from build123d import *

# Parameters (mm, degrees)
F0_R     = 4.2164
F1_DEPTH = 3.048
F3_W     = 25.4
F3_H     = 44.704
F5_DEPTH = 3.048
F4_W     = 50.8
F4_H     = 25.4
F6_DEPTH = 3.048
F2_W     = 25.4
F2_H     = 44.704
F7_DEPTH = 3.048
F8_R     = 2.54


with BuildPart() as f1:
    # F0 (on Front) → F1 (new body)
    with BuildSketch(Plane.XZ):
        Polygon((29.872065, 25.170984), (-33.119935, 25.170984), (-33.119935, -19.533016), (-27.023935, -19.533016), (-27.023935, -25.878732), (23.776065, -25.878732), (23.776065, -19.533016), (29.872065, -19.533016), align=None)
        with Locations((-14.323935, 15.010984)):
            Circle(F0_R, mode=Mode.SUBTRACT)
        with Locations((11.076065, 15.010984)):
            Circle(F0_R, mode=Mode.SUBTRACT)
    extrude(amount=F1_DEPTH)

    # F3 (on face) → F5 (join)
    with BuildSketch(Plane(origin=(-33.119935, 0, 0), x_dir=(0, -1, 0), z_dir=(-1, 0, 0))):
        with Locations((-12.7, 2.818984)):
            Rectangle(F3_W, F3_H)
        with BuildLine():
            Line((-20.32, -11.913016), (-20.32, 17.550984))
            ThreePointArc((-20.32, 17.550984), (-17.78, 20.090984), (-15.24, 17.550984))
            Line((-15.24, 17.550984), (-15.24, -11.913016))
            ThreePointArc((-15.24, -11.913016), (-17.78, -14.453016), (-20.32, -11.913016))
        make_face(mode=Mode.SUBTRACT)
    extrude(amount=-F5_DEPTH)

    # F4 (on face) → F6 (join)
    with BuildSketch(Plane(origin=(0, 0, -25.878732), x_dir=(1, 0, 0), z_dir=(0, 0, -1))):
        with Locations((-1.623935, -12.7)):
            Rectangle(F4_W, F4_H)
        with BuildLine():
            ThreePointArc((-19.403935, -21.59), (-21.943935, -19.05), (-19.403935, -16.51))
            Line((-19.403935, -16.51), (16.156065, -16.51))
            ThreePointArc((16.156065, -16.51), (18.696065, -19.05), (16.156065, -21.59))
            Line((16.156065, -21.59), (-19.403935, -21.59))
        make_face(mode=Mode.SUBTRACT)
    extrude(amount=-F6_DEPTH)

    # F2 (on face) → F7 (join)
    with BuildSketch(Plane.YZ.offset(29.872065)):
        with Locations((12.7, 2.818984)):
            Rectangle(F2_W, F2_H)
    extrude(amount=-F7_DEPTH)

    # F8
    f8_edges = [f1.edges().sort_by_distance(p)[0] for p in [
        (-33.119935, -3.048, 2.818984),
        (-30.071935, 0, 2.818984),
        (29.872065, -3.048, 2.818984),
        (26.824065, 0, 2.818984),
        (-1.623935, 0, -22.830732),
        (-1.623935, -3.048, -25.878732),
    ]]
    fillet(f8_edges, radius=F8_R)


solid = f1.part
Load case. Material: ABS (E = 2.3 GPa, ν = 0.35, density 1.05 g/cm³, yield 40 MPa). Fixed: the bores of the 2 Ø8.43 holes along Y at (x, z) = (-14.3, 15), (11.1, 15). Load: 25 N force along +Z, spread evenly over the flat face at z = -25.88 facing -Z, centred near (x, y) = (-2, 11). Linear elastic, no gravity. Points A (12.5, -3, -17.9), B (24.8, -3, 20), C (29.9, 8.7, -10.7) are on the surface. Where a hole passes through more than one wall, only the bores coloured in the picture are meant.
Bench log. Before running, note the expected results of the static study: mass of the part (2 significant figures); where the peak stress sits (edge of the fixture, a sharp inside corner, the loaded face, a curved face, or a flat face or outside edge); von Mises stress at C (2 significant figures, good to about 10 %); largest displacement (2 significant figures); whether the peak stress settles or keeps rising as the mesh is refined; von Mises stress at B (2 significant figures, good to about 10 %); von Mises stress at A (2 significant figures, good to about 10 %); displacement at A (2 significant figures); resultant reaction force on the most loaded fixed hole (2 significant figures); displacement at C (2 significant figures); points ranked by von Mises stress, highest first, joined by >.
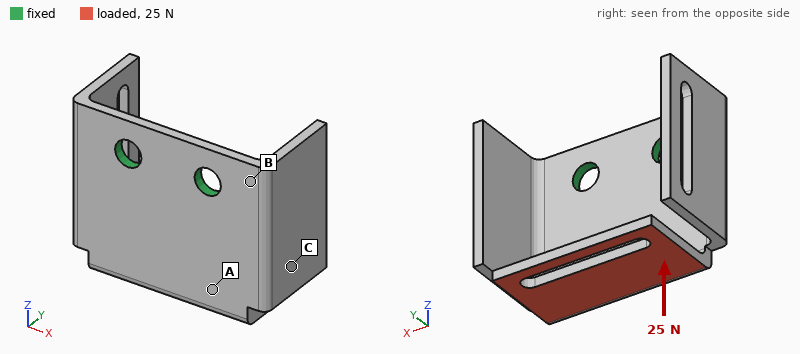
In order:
20 g
a sharp inside corner
0.42 MPa
0.87 mm
keeps rising
1.5 MPa
2.9 MPa
0.21 mm
13 N
0.16 mm
A > B > C
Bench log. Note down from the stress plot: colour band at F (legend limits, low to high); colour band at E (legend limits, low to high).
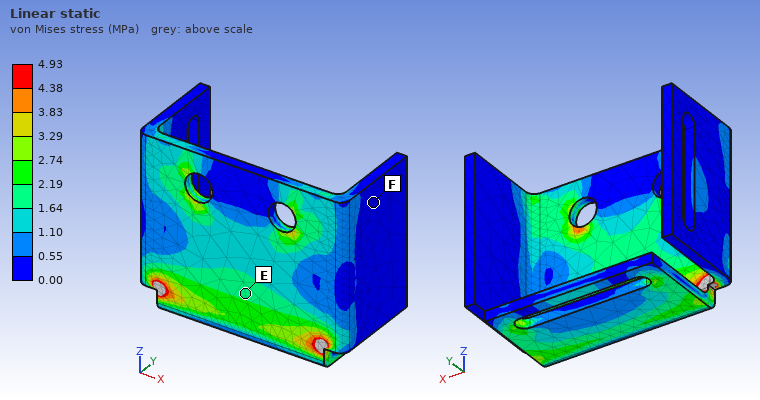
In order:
0.00 to 0.55 MPa
1.64 to 2.19 MPa
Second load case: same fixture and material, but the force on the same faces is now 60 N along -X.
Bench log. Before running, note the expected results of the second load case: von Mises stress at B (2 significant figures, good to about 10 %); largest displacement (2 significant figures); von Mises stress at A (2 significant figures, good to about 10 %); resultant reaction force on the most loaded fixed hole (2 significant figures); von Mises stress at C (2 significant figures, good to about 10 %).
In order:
4.5 MPa
0.91 mm
2.3 MPa
81 N
0.76 MPa
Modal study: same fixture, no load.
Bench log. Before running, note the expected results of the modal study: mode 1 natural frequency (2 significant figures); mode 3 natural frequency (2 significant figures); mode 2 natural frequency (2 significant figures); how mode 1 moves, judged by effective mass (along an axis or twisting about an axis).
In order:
330 Hz
610 Hz
410 Hz
along Y
